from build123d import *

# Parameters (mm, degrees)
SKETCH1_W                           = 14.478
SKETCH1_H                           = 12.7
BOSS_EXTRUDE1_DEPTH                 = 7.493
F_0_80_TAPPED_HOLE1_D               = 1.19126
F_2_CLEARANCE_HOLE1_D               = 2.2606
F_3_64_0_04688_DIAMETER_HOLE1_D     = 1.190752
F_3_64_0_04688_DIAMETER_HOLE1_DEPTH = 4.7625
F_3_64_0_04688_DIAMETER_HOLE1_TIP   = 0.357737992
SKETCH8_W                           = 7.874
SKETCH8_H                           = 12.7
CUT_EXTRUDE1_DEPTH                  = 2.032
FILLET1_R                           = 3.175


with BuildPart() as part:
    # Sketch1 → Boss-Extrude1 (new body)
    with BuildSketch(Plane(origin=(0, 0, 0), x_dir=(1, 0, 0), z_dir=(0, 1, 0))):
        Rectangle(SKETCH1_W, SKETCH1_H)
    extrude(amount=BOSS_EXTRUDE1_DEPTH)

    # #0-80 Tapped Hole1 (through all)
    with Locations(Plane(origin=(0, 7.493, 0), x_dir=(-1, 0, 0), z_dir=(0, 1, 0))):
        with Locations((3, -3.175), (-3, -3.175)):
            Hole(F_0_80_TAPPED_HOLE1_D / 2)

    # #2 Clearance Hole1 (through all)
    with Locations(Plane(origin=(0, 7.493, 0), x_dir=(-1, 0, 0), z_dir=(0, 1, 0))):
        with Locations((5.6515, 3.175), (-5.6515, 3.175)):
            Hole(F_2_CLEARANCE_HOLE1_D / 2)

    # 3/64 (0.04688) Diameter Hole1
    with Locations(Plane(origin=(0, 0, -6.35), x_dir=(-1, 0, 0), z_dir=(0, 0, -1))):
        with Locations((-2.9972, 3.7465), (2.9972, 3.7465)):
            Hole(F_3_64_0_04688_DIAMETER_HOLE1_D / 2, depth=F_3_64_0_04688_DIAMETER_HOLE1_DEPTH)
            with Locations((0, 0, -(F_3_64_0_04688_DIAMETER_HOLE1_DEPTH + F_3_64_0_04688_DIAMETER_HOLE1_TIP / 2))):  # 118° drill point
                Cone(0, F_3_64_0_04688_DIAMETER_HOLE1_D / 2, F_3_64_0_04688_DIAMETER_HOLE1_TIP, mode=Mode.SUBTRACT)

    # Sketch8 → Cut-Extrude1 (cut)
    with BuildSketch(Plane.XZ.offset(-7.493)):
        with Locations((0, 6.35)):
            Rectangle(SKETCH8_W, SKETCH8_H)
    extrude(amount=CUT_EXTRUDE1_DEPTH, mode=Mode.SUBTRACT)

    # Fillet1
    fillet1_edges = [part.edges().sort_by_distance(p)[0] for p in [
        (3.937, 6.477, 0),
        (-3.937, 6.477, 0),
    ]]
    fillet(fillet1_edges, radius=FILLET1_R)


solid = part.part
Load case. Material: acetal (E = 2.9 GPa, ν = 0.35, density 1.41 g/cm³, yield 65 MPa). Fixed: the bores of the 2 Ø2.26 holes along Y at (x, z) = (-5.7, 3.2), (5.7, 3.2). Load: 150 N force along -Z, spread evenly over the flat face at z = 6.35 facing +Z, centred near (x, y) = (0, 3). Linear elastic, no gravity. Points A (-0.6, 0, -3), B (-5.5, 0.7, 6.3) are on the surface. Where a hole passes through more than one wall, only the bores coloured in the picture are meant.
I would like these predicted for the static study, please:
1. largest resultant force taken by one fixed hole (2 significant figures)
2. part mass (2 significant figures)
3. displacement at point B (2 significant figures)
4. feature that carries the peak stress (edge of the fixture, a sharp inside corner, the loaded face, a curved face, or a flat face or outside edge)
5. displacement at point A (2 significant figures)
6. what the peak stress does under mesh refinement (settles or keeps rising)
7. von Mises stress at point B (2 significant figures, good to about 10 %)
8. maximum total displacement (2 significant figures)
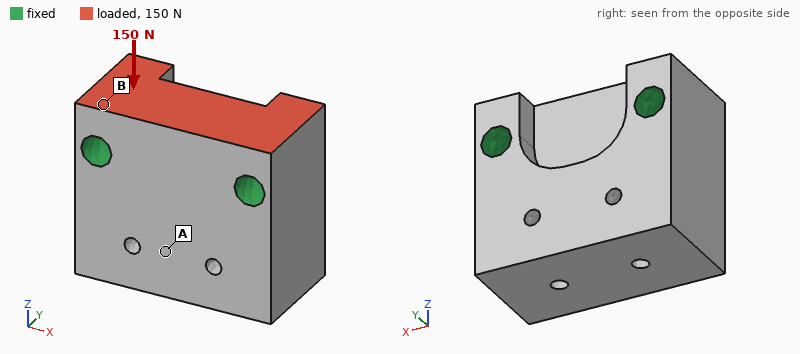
75 N
1.7 g
1.6 µm
edge of the fixture
2.1 µm
keeps rising
2.1 MPa
5.0 µm
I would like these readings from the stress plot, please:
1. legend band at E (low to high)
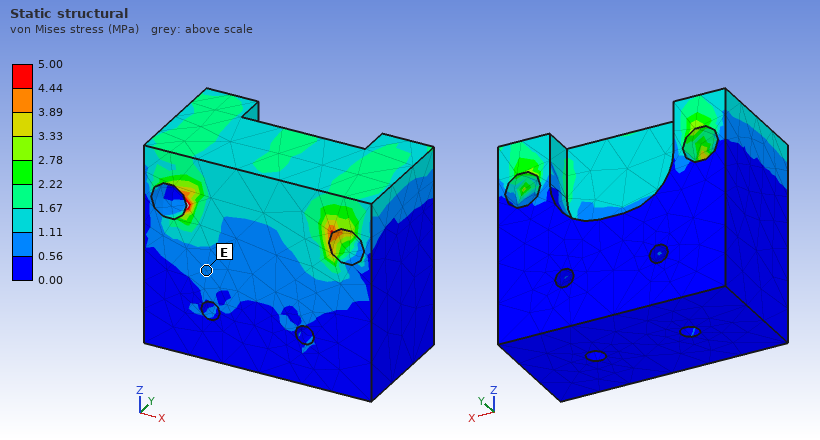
0.56 to 1.11 MPa
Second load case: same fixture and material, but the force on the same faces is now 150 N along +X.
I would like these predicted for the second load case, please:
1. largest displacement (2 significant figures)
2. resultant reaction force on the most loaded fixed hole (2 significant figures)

8.5 µm
80 N
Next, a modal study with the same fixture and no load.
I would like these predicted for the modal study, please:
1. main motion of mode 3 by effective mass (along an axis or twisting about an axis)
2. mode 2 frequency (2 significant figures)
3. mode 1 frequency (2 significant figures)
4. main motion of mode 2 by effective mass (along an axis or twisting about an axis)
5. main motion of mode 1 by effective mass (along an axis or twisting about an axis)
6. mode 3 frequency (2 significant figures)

along X
18 kHz
13 kHz
along X
along Y
20 kHz
